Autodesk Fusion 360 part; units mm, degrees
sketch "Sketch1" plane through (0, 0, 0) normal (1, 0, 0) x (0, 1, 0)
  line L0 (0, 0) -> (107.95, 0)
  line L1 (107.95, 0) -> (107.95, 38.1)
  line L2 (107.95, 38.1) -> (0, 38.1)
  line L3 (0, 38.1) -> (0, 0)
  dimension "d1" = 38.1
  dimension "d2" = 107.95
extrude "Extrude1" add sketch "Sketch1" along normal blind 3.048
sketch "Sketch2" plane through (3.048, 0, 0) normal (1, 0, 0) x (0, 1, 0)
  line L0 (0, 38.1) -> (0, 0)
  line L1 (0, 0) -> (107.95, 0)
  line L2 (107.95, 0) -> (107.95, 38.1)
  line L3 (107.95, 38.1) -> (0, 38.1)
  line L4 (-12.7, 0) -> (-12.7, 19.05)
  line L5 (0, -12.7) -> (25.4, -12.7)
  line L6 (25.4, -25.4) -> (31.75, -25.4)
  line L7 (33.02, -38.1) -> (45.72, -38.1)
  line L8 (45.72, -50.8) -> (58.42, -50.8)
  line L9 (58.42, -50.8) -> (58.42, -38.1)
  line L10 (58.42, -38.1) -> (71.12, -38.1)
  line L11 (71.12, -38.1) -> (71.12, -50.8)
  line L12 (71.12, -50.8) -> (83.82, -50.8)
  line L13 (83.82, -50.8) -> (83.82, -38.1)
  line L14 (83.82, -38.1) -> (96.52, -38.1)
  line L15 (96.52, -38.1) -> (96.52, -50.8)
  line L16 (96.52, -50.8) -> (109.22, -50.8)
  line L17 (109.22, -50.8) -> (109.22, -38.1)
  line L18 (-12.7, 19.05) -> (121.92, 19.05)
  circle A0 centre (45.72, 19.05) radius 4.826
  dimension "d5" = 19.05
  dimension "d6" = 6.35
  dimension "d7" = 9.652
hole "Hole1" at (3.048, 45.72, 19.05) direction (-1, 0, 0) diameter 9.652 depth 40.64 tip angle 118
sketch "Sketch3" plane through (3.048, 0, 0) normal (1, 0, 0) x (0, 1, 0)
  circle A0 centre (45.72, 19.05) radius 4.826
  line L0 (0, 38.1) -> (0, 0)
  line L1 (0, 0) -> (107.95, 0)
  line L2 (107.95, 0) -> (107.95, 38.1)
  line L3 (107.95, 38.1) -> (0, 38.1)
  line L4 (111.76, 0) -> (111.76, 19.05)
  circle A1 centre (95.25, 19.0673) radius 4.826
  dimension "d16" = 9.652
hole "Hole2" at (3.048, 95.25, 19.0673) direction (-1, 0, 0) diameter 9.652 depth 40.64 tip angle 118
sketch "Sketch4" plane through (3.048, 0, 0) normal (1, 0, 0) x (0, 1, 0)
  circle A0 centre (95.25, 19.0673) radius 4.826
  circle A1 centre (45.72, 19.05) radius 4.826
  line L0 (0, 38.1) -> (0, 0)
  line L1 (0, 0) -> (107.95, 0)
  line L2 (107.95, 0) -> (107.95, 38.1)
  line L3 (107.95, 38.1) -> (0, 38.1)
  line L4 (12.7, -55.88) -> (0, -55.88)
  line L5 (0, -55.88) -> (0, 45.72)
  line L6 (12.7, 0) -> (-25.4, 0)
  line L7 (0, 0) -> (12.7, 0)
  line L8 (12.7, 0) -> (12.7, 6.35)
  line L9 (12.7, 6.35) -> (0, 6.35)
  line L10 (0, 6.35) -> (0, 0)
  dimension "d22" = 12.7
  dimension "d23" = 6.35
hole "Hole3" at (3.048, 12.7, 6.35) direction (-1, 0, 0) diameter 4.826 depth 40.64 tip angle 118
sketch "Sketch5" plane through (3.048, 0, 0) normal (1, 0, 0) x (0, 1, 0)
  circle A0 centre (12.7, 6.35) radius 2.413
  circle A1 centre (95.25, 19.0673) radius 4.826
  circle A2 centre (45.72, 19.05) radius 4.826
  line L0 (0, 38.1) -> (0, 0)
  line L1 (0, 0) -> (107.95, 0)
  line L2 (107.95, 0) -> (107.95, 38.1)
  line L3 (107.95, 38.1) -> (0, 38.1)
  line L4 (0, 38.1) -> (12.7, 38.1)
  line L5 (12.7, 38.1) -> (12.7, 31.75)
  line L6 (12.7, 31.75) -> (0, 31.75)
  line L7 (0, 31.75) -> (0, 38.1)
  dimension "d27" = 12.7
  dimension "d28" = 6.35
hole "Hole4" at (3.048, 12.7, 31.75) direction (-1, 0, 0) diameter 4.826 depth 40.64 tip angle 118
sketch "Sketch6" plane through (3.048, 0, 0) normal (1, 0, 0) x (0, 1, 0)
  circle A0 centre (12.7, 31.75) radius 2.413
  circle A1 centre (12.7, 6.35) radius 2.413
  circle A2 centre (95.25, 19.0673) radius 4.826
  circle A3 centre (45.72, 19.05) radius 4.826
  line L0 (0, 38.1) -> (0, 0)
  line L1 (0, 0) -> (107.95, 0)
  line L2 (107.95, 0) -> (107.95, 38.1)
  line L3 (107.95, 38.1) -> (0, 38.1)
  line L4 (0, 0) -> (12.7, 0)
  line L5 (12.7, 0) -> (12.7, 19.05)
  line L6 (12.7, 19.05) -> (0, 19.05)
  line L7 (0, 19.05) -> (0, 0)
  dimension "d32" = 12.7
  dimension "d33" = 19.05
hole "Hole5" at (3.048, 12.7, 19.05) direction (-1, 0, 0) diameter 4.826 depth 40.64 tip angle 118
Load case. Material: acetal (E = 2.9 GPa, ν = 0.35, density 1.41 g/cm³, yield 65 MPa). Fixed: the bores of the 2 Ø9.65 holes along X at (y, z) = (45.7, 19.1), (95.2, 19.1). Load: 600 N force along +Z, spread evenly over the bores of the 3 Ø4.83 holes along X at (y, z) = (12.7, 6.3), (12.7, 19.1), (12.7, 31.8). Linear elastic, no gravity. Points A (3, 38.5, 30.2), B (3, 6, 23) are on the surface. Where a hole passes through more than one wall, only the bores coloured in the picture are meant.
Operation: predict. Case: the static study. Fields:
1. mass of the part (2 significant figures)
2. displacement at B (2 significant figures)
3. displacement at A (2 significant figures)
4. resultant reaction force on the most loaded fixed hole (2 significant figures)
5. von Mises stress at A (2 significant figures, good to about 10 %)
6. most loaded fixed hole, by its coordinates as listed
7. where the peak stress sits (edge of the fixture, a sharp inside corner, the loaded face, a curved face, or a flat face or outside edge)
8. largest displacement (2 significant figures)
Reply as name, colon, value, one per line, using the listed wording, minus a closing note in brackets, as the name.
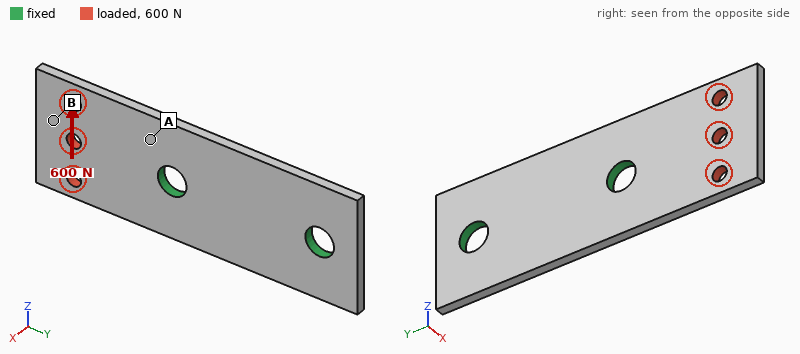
mass of the part: 17 g
displacement at B: 0.69 mm
displacement at A: 0.14 mm
resultant reaction force on the most loaded fixed hole: 840 N
von Mises stress at A: 14 MPa
most loaded fixed hole, by its coordinates as listed: (45.7, 19.1)
where the peak stress sits: edge of the fixture
largest displacement: 0.84 mm
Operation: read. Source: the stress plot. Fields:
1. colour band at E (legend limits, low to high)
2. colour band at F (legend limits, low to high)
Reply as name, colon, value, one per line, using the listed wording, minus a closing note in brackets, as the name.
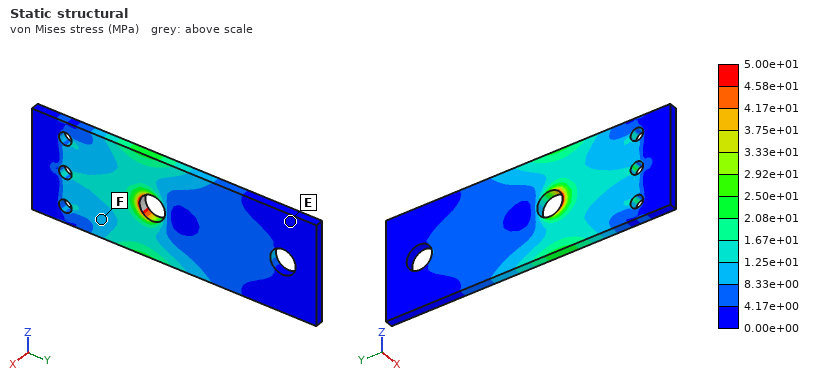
colour band at E: 0.00e+00 to 4.17e+00 MPa
colour band at F: 8.33e+00 to 1.25e+01 MPa
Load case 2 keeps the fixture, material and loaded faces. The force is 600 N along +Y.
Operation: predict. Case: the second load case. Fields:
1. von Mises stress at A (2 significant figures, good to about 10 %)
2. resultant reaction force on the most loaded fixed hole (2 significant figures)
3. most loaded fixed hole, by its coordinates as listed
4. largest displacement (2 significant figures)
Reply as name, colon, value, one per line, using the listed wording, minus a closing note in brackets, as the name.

von Mises stress at A: 3.9 MPa
resultant reaction force on the most loaded fixed hole: 530 N
most loaded fixed hole, by its coordinates as listed: (45.7, 19.1)
largest displacement: 79 µm
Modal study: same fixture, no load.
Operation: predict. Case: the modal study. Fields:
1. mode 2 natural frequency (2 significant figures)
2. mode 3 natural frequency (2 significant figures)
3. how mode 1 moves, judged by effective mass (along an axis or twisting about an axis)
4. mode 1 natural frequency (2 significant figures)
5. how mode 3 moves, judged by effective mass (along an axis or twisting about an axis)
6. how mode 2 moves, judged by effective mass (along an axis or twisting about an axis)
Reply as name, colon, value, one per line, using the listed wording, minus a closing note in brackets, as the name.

mode 2 natural frequency: 850 Hz
mode 3 natural frequency: 1800 Hz
how mode 1 moves, judged by effective mass: along X
mode 1 natural frequency: 390 Hz
how mode 3 moves, judged by effective mass: twisting about Y
how mode 2 moves, judged by effective mass: twisting about Y
